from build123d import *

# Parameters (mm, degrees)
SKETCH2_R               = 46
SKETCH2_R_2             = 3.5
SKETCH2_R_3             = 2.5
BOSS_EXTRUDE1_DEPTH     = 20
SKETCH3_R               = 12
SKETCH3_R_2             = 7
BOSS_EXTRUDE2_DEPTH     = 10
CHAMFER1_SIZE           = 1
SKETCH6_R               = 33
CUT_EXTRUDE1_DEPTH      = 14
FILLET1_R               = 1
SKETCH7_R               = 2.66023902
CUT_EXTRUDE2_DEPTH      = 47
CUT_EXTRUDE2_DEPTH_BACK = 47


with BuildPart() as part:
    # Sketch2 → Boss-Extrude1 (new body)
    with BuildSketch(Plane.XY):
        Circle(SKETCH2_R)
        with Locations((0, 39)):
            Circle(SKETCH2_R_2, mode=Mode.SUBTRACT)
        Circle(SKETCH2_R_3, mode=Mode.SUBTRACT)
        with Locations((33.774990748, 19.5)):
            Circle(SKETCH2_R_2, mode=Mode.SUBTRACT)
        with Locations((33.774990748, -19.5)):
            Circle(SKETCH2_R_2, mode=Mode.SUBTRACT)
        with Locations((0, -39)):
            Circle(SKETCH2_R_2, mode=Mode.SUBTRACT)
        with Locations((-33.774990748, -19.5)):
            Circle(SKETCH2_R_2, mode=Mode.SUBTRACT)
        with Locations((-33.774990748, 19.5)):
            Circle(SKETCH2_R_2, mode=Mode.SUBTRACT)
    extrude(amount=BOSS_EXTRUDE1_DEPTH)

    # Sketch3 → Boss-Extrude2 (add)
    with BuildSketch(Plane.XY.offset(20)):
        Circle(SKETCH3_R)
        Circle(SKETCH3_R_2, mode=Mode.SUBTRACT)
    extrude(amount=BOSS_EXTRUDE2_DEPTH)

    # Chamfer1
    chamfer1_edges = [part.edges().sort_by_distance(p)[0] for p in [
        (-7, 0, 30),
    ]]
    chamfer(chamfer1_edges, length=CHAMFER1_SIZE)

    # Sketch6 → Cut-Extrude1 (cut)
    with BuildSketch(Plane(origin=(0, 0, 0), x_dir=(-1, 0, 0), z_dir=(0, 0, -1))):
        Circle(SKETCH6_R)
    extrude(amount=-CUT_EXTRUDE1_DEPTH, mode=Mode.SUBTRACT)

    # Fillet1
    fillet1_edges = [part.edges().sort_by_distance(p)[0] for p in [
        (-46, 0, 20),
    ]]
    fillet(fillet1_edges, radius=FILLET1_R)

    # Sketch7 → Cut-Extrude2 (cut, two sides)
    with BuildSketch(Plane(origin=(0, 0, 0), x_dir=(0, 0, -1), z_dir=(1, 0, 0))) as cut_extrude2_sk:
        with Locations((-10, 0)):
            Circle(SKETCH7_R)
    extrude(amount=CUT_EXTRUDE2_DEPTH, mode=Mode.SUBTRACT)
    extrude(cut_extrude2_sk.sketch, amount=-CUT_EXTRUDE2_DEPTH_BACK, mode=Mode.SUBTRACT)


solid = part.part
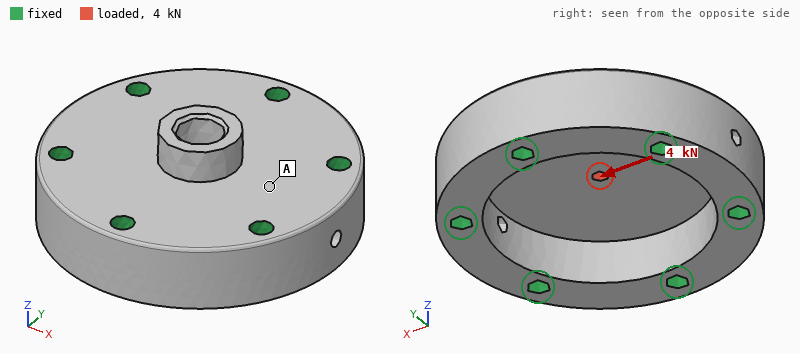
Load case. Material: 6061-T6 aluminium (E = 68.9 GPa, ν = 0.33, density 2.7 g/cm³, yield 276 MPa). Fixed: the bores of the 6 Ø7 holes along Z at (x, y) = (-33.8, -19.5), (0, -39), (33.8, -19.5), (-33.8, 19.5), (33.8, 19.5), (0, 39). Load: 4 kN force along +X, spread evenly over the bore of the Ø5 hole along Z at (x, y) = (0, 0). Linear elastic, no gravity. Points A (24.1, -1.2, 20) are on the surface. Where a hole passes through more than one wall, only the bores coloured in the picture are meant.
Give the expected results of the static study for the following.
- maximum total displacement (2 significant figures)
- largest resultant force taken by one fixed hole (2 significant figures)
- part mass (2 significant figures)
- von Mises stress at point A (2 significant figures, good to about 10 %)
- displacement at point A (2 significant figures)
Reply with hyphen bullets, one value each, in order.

- 7.5 µm
- 900 N
- 220 g
- 5.3 MPa
- 2.2 µm
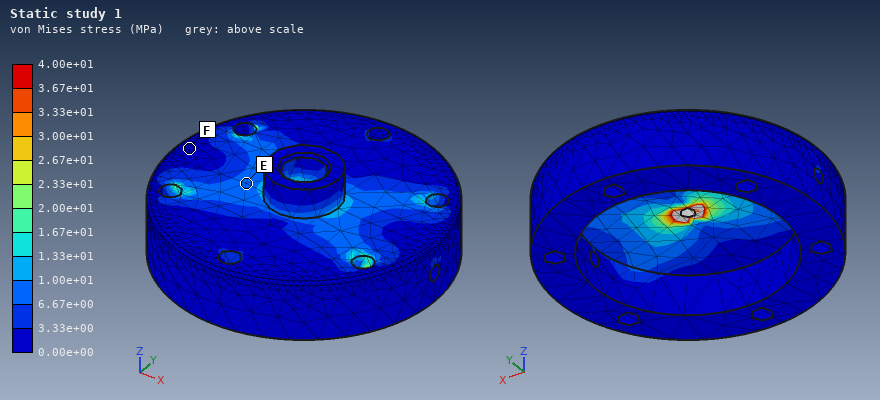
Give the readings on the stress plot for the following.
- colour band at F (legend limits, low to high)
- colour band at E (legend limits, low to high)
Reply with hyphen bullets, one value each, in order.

- 0.00e+00 to 3.33e+00 MPa
- 6.67e+00 to 1.00e+01 MPa
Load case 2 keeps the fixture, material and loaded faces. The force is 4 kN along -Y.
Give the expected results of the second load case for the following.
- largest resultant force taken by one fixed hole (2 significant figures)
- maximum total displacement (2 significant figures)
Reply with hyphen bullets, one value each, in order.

- 1.0 kN
- 7.5 µm
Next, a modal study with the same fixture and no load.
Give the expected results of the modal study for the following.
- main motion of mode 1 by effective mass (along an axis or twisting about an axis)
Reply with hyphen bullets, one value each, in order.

- along Z
